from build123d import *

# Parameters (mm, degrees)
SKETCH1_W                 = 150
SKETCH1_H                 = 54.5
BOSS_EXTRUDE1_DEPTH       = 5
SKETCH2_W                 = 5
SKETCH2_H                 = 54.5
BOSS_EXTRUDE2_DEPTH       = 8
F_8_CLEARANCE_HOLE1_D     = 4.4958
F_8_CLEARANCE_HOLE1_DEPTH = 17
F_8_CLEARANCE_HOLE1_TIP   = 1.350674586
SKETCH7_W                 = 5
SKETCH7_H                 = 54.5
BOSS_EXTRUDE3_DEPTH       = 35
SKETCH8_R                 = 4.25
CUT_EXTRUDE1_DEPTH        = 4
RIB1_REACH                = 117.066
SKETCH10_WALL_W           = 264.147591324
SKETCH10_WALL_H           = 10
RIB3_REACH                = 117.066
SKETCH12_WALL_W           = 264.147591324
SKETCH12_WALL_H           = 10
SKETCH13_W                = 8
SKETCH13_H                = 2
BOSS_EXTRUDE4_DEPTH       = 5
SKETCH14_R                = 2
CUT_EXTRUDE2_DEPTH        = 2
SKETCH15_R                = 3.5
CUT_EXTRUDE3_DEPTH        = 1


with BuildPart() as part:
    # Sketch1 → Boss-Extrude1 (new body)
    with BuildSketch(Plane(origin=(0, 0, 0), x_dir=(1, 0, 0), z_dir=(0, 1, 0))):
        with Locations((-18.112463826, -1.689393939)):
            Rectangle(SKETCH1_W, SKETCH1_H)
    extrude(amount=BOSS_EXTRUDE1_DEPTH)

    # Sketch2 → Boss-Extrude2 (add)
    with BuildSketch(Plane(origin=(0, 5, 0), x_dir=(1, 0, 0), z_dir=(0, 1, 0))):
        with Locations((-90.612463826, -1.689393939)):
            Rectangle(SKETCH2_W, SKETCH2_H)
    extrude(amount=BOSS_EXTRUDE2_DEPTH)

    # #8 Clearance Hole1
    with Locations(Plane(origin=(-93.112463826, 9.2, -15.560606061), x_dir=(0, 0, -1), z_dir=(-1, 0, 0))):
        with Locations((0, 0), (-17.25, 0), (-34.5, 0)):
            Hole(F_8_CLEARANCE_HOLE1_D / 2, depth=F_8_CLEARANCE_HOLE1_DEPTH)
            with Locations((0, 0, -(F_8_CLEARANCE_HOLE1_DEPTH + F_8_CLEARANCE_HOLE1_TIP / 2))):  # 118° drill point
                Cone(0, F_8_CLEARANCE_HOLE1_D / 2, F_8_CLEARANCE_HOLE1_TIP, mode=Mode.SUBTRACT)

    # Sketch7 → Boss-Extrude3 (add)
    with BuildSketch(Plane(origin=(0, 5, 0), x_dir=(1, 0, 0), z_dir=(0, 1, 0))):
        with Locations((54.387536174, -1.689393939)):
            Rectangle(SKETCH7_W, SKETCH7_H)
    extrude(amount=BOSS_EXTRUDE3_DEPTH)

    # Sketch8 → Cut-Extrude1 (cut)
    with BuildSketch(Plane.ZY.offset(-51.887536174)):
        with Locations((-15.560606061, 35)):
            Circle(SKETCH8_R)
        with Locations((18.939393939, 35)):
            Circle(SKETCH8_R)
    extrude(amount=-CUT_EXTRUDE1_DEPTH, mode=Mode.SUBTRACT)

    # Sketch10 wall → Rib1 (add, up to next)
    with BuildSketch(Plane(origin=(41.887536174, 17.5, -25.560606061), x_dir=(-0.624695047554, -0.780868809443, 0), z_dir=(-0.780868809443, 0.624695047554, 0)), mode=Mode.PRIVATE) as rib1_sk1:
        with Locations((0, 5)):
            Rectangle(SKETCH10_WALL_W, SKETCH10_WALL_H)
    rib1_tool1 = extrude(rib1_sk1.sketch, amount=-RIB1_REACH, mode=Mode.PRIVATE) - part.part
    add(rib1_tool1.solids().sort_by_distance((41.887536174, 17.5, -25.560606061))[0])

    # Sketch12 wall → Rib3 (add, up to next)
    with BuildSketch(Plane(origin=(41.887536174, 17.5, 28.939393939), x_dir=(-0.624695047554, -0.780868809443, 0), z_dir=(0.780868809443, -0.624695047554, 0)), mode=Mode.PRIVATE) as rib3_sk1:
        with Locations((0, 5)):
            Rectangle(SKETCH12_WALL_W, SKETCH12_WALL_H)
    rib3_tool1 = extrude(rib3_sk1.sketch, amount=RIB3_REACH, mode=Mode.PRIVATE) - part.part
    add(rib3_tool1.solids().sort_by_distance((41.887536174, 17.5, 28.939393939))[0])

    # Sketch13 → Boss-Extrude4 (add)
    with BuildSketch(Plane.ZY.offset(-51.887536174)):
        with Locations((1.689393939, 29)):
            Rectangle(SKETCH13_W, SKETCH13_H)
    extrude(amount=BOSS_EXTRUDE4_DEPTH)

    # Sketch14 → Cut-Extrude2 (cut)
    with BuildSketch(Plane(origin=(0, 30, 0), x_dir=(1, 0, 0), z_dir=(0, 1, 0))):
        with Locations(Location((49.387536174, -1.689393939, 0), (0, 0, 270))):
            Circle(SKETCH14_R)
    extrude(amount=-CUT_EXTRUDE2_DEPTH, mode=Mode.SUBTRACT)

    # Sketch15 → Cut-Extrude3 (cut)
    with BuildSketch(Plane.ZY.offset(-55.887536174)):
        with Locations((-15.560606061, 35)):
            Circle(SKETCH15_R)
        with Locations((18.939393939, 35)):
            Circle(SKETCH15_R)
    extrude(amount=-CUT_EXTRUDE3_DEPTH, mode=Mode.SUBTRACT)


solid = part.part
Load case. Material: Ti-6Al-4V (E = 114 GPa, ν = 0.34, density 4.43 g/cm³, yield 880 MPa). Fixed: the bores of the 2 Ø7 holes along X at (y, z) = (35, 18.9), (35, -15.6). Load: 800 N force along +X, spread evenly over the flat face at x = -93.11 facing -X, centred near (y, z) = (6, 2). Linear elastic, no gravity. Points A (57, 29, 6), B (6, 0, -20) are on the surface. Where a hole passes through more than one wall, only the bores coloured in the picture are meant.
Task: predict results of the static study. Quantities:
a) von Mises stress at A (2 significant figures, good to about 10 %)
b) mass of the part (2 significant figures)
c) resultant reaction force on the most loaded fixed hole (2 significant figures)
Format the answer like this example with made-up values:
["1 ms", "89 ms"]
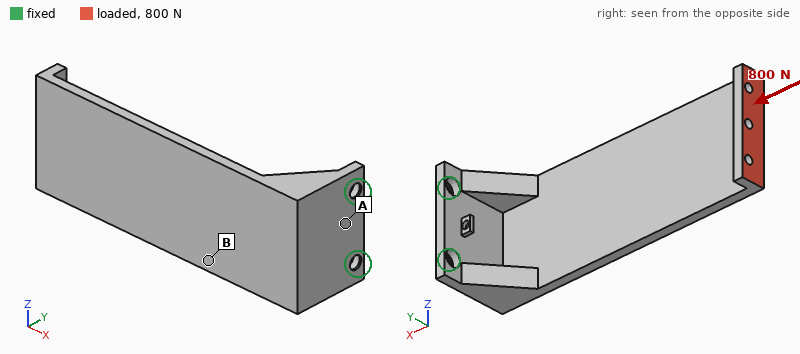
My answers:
["43 MPa", "250 g", "410 N"]
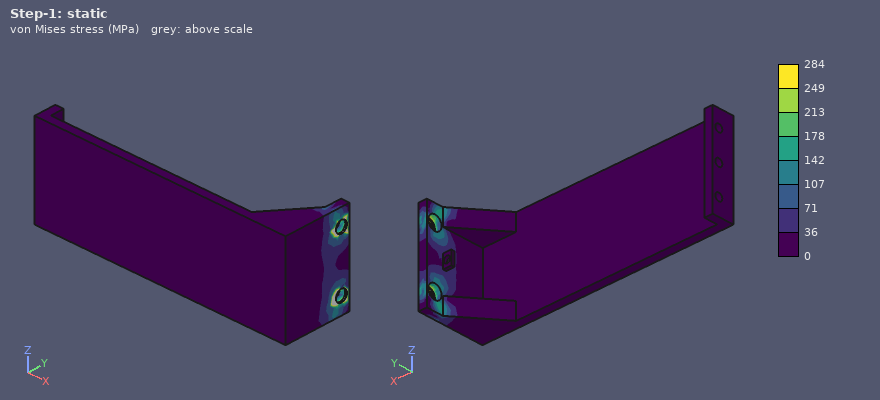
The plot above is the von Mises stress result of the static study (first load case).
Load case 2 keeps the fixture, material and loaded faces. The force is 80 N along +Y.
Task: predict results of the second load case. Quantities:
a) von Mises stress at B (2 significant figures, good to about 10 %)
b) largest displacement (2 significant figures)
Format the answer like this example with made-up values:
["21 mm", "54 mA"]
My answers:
["35 MPa", "1.6 mm"]
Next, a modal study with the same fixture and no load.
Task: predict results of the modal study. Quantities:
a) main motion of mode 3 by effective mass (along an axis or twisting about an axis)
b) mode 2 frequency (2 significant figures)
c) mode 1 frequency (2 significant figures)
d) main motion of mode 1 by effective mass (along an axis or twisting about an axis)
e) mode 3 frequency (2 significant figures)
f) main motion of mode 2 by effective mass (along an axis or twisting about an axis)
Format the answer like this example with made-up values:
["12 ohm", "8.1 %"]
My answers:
["along X", "420 Hz", "150 Hz", "along Y", "680 Hz", "along Z"]
